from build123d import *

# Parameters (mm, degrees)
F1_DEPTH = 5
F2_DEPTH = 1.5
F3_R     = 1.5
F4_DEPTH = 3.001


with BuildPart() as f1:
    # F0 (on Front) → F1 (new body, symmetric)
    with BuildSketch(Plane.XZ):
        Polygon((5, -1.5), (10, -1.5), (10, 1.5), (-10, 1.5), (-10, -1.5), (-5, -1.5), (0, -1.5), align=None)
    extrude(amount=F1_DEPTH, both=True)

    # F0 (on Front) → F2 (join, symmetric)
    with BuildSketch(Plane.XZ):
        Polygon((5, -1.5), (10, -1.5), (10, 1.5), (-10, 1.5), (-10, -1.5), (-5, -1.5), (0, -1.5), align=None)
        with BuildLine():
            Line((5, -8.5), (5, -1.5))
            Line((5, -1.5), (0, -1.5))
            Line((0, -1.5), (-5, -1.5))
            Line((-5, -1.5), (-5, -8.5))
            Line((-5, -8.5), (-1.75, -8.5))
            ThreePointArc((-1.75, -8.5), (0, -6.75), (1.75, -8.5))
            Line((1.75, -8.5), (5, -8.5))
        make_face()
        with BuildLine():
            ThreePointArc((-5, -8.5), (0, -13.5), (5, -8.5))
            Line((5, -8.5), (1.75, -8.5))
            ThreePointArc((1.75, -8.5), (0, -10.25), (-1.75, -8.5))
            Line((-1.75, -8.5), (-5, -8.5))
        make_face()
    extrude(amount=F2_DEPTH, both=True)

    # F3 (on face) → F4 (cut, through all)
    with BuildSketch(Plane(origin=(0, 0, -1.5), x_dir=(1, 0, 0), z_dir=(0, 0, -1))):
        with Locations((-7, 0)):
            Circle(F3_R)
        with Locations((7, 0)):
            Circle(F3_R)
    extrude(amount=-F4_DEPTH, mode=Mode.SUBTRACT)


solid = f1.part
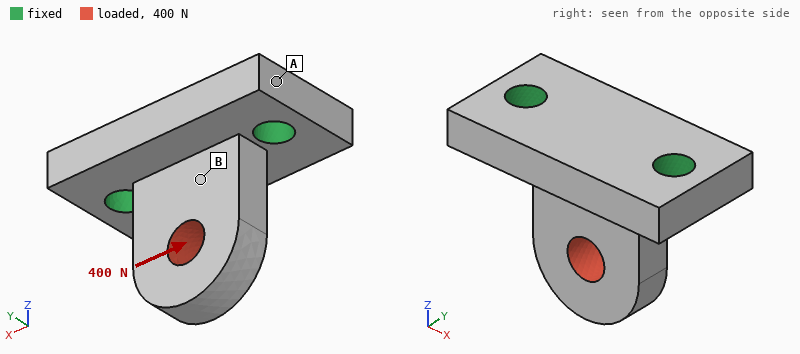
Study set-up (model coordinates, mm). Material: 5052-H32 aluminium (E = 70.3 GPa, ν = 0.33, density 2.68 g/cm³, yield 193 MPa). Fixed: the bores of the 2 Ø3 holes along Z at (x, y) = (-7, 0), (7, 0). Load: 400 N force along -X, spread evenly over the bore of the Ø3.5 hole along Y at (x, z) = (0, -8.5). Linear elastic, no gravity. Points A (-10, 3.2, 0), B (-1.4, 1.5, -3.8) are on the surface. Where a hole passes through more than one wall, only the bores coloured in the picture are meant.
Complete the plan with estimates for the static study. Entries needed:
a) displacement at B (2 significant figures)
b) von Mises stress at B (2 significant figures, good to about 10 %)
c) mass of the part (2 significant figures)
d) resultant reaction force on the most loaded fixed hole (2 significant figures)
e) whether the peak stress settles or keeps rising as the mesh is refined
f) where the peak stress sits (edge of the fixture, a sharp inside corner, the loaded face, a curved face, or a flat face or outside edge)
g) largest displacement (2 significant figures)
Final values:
3.2 µm
31 MPa
2.3 g
360 N
keeps rising
a sharp inside corner
16 µm
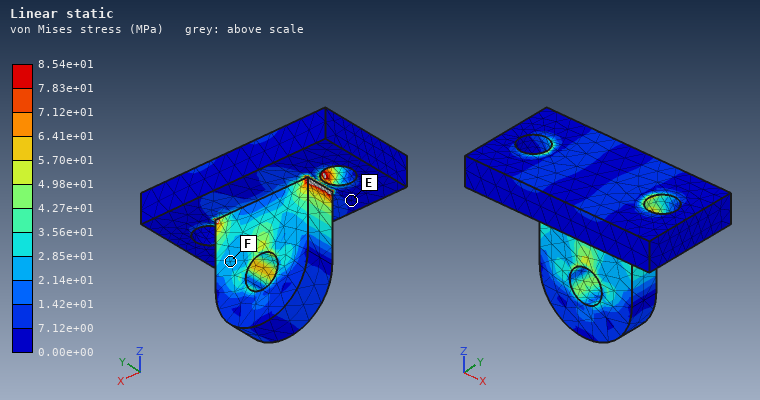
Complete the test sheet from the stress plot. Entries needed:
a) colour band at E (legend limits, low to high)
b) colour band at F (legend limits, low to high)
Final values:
0.00e+00 to 7.12e+00 MPa
2.14e+01 to 2.85e+01 MPa
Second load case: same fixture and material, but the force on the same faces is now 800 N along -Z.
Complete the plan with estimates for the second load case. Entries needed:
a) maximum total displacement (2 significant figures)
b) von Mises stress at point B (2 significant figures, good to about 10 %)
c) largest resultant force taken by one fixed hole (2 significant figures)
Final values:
7.9 µm
20 MPa
420 N
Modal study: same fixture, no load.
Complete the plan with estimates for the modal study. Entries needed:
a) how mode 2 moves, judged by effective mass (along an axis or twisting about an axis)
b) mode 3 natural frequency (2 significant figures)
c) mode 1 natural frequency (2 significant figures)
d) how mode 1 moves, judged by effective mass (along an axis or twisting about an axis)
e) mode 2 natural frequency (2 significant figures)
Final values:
along X
42 kHz
15 kHz
along Y
37 kHz
